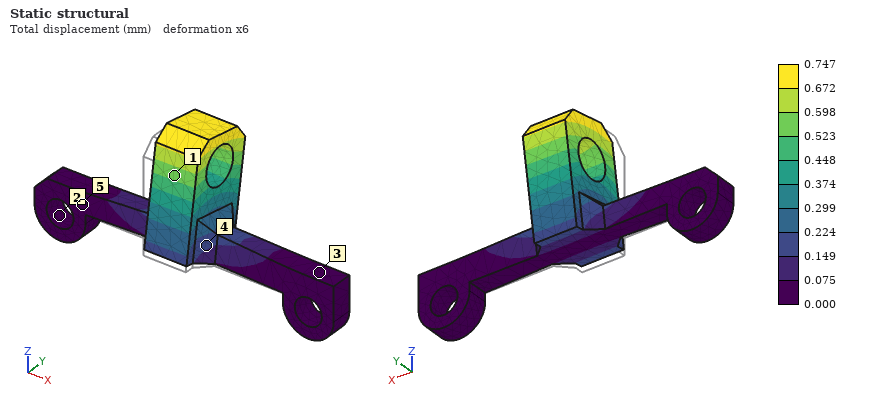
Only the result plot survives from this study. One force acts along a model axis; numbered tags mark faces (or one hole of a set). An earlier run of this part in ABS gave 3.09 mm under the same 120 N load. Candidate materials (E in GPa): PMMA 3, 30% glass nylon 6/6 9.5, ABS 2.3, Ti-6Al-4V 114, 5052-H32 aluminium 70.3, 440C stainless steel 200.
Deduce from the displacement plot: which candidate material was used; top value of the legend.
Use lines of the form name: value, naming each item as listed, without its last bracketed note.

which candidate material was used: 30% glass nylon 6/6
top value of the legend: 0.747 mm
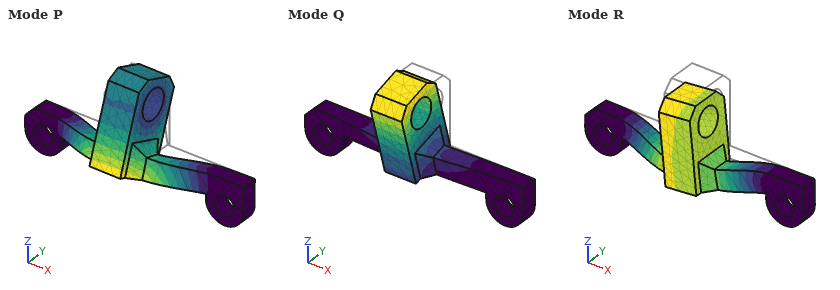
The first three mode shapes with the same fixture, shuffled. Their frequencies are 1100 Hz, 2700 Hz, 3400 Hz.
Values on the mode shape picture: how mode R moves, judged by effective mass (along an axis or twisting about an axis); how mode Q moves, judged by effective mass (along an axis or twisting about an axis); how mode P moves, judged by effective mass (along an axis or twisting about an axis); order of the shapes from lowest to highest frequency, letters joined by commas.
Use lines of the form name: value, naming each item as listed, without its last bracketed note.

how mode R moves, judged by effective mass: along Z
how mode Q moves, judged by effective mass: along Y
how mode P moves, judged by effective mass: along Y
order of the shapes from lowest to highest frequency, letters joined by commas: Q, R, P
